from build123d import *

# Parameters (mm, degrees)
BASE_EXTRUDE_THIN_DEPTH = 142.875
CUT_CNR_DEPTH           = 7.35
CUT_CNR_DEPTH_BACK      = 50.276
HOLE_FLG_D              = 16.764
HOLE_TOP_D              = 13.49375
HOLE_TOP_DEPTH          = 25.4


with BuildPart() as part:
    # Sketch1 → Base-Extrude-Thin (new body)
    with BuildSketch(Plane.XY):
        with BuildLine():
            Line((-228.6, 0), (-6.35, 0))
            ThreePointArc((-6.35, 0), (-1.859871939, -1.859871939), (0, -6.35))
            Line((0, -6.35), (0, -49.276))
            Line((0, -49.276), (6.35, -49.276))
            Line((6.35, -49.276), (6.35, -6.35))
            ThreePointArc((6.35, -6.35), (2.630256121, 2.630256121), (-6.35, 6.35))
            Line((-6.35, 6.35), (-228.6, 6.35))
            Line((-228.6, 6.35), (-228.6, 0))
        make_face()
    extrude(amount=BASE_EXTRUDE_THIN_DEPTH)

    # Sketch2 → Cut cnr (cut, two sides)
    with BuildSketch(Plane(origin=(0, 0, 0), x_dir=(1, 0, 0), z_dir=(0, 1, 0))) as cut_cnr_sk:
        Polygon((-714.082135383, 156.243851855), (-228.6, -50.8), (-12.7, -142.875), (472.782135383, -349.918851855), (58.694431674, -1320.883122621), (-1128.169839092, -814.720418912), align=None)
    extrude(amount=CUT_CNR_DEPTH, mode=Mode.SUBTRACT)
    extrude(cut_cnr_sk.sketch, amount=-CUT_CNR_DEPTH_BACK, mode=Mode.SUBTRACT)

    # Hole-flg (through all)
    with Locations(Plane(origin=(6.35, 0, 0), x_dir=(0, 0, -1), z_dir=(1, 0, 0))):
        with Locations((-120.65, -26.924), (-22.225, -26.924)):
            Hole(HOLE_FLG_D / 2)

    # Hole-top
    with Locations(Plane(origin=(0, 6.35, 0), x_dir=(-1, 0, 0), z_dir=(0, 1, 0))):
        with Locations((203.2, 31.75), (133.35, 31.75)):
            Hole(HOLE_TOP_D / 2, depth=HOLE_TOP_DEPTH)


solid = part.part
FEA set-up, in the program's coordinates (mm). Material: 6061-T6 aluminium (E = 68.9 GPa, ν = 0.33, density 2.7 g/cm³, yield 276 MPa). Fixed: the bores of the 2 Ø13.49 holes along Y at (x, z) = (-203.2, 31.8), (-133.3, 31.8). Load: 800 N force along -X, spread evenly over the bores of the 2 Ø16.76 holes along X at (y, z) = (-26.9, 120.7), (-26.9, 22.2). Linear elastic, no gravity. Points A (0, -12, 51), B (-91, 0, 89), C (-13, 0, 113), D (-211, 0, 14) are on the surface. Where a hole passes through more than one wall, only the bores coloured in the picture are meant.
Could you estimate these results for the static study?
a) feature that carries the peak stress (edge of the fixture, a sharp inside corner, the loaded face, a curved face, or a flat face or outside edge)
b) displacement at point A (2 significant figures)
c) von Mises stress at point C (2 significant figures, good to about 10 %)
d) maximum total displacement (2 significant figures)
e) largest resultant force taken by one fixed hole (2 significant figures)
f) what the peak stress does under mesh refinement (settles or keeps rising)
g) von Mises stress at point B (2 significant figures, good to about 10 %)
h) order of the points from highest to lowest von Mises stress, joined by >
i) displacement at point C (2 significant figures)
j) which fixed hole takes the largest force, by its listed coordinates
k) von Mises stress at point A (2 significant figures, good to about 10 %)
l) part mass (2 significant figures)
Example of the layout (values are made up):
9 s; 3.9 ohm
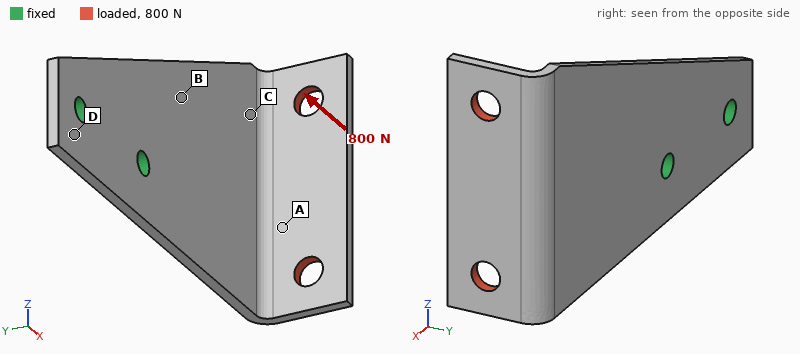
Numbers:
edge of the fixture; 1.4 mm; 24 MPa; 2.0 mm; 640 N; keeps rising; 33 MPa; B > C > A > D; 1.2 mm; (-133.3, 31.8); 13 MPa; 500 g
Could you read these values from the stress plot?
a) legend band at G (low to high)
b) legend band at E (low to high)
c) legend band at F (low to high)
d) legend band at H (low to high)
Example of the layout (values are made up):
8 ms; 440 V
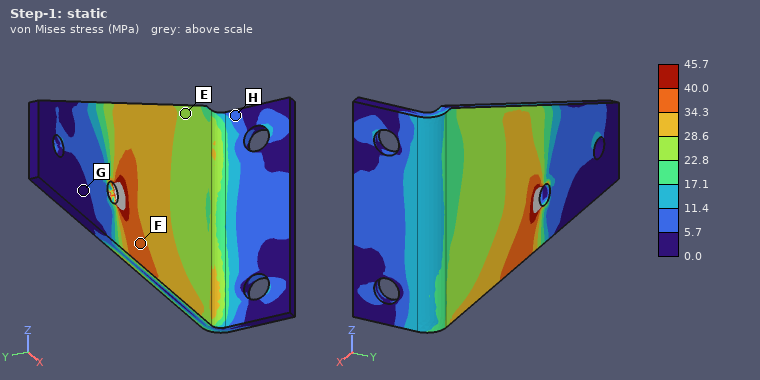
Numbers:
0.0 to 5.7 MPa; 22.8 to 28.6 MPa; 34.3 to 40.0 MPa; 5.7 to 11.4 MPa
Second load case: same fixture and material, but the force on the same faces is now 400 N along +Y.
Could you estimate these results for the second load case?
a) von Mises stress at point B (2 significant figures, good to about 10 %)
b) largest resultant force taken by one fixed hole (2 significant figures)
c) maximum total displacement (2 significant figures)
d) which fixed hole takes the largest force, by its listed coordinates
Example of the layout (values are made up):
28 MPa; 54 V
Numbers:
44 MPa; 620 N; 3.3 mm; (-133.3, 31.8)
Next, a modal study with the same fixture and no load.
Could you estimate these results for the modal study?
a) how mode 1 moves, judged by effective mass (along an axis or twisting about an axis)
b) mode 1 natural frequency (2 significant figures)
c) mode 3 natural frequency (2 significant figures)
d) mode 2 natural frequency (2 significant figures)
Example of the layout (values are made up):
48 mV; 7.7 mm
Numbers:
along Y; 140 Hz; 770 Hz; 320 Hz
